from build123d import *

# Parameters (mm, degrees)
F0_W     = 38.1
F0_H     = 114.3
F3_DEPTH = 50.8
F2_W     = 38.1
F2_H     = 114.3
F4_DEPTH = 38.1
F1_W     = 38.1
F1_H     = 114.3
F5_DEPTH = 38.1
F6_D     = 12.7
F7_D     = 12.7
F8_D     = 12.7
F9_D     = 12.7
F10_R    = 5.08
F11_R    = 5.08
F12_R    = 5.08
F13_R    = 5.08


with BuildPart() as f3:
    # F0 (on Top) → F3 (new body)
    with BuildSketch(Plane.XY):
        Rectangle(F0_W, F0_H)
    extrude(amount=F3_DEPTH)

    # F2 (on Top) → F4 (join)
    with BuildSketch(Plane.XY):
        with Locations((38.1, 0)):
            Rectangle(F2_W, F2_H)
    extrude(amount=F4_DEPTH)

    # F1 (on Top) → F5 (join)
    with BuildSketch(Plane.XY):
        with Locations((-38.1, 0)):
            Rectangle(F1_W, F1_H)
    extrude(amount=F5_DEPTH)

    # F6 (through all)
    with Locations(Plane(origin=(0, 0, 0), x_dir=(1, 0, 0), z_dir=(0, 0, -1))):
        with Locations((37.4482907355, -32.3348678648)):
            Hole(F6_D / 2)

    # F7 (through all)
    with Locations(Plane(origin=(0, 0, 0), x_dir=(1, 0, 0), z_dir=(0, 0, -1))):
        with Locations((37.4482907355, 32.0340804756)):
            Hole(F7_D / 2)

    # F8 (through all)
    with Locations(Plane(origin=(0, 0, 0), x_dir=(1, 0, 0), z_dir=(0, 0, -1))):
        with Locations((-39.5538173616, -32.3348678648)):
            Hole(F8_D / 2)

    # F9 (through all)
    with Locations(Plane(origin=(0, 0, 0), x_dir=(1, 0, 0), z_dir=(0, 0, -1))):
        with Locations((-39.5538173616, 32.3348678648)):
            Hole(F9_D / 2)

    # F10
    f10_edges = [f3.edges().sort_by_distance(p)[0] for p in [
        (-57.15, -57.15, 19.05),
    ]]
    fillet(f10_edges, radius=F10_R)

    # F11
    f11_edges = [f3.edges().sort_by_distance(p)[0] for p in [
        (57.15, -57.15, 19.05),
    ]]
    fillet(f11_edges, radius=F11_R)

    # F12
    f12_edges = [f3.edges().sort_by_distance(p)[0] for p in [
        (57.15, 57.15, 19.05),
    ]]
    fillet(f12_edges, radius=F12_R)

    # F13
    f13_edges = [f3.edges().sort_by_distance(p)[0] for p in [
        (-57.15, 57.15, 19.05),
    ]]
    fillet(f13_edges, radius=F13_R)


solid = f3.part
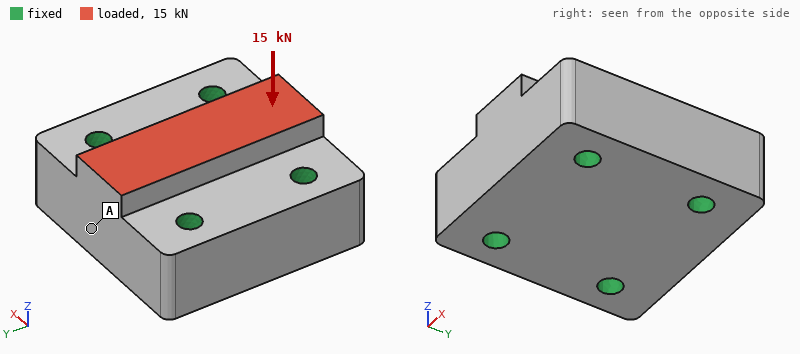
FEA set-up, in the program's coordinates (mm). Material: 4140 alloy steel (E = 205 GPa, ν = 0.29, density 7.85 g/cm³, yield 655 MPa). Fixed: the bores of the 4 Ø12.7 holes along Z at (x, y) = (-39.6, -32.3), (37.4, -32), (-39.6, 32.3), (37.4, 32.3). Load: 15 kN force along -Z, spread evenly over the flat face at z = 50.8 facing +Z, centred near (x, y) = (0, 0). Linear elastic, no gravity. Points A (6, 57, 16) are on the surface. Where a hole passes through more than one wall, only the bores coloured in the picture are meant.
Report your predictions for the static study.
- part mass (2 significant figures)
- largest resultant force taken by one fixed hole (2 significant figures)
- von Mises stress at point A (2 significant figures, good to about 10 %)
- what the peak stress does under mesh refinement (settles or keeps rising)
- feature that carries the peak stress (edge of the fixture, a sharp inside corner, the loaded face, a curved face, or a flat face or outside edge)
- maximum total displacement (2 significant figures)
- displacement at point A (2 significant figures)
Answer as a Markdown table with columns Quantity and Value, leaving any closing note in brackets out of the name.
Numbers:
| Quantity | Value |
|---|---|
| part mass | 4.2 kg |
| largest resultant force taken by one fixed hole | 4.0 kN |
| von Mises stress at point A | 1.7 MPa |
| what the peak stress does under mesh refinement | keeps rising |
| feature that carries the peak stress | edge of the fixture |
| maximum total displacement | 1.4 µm |
| displacement at point A | 0.96 µm |
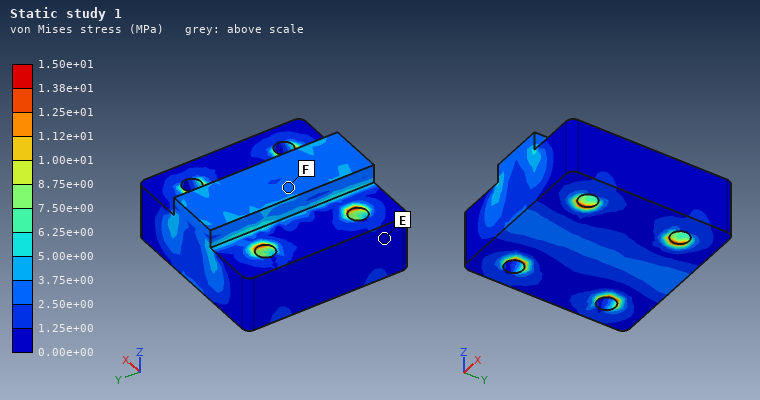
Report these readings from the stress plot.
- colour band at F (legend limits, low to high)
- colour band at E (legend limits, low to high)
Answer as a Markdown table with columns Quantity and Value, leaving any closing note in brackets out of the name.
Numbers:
| Quantity | Value |
|---|---|
| colour band at F | 2.50e+00 to 3.75e+00 MPa |
| colour band at E | 0.00e+00 to 1.25e+00 MPa |
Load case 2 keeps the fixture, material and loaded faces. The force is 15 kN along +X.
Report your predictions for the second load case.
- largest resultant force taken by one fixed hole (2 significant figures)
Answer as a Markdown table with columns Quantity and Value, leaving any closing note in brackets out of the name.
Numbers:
| Quantity | Value |
|---|---|
| largest resultant force taken by one fixed hole | 4.9 kN |
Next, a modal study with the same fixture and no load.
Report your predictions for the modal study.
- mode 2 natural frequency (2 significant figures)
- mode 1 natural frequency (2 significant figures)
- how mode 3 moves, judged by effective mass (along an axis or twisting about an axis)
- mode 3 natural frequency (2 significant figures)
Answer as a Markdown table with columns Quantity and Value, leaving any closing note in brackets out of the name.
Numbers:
| Quantity | Value |
|---|---|
| mode 2 natural frequency | 14 kHz |
| mode 1 natural frequency | 14 kHz |
| how mode 3 moves, judged by effective mass | along Y |
| mode 3 natural frequency | 17 kHz |
